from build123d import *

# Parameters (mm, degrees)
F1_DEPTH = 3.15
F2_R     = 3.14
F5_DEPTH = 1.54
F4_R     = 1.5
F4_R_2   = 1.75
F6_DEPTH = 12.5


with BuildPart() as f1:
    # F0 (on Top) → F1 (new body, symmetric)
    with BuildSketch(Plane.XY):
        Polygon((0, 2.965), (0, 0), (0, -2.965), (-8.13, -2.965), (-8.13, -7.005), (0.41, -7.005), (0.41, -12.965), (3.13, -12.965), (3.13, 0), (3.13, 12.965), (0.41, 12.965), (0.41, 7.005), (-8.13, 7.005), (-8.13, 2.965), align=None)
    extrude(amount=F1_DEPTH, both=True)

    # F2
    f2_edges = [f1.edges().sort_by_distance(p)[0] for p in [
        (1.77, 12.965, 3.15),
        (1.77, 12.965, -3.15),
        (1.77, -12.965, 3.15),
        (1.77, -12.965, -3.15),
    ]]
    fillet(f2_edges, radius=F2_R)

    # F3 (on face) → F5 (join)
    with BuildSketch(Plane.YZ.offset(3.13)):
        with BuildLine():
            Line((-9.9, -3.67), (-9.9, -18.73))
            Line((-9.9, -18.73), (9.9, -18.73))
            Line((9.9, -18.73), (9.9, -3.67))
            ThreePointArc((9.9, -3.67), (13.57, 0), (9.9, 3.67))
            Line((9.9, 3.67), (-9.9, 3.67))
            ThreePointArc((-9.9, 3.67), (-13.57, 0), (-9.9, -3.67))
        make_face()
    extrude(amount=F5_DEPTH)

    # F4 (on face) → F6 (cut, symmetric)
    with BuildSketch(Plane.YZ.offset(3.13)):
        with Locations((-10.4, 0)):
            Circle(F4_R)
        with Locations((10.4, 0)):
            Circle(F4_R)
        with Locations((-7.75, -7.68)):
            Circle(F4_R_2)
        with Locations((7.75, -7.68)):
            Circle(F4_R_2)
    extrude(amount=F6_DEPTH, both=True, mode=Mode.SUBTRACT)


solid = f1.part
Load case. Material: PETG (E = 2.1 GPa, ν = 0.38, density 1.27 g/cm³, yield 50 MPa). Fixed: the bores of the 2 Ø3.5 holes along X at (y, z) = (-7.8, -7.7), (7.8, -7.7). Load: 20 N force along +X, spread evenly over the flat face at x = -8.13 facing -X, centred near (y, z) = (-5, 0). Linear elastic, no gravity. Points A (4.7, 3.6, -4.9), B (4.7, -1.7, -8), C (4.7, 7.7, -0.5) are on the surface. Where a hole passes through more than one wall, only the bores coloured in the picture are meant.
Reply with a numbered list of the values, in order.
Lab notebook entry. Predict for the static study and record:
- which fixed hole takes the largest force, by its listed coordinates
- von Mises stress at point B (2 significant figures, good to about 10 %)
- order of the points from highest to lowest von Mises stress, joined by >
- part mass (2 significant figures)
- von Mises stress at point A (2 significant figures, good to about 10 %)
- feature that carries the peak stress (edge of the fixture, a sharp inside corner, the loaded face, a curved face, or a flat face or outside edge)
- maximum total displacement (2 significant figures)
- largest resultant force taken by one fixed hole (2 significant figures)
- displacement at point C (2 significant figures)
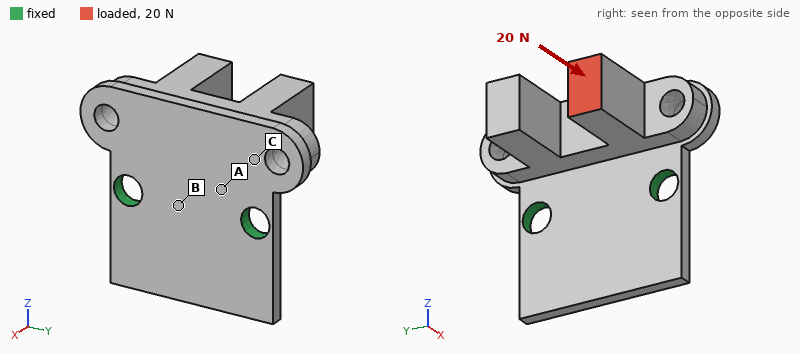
1. (-7.8, -7.7)
2. 3.8 MPa
3. A > B > C
4. 1.9 g
5. 7.9 MPa
6. a flat face or outside edge
7. 0.45 mm
8. 17 N
9. 0.12 mm
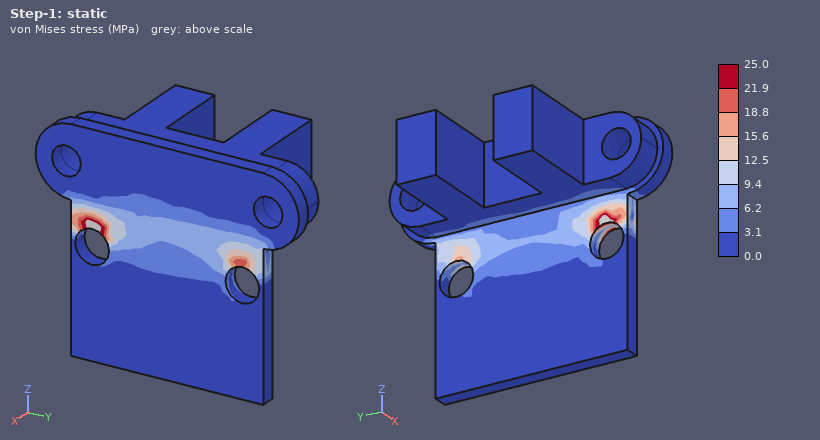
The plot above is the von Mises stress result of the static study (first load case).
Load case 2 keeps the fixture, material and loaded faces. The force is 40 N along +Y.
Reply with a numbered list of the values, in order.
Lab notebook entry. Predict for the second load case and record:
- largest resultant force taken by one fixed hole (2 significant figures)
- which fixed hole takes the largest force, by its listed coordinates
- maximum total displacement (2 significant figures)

1. 44 N
2. (7.8, -7.7)
3. 0.39 mm
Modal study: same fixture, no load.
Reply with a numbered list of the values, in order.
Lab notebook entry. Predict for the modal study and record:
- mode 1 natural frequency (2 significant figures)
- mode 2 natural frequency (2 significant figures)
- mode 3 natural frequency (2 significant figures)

1. 1000 Hz
2. 3000 Hz
3. 3100 Hz
